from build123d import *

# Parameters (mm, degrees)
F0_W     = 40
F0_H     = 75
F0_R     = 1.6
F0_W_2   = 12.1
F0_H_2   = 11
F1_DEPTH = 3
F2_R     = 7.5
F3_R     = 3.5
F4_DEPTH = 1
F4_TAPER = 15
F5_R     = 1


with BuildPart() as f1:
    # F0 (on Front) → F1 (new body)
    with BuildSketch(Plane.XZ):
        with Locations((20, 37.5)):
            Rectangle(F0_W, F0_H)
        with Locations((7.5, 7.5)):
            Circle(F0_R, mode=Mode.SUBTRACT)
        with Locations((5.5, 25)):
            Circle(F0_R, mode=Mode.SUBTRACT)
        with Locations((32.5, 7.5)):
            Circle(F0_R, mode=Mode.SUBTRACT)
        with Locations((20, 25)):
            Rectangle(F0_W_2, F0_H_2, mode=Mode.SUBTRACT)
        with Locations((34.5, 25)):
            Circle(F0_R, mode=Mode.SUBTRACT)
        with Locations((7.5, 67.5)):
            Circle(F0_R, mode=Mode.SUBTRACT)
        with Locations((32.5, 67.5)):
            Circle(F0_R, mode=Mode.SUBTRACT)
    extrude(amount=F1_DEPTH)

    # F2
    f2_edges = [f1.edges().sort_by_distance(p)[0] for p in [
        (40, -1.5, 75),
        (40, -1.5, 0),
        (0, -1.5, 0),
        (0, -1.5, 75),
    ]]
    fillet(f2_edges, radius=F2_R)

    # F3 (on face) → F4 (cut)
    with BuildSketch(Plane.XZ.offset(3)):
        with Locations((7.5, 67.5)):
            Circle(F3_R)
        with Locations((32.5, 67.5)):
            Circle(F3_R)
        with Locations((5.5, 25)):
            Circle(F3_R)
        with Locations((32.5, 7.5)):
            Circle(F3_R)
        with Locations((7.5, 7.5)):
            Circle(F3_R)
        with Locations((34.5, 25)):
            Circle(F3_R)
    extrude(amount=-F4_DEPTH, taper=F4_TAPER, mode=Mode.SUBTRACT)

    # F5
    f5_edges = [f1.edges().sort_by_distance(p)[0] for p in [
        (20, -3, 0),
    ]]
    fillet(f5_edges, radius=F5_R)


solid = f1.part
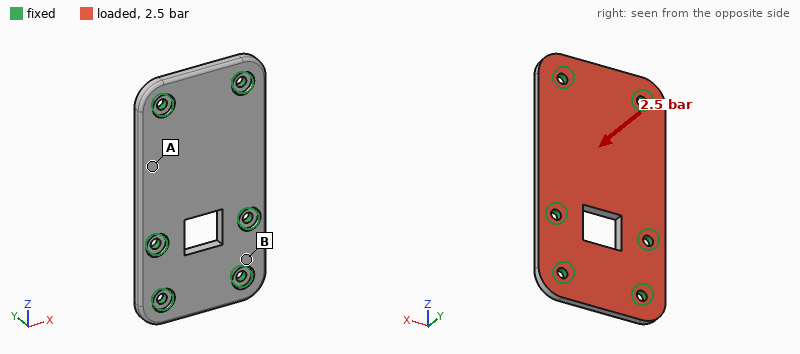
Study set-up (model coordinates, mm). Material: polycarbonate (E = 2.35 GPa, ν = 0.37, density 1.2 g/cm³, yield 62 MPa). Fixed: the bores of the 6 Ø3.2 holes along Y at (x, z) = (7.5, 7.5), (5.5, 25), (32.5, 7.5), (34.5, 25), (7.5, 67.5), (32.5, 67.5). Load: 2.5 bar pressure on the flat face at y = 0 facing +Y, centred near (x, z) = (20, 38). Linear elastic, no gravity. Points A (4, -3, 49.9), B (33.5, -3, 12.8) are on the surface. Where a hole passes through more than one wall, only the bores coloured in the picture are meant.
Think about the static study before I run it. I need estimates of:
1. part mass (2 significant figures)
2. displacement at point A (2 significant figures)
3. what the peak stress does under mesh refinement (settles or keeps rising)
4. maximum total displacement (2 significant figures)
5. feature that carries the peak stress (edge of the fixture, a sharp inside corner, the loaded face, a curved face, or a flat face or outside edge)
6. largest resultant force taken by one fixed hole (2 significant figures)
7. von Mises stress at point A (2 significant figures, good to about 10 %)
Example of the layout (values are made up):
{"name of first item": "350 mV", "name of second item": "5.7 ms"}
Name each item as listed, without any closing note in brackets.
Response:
{"part mass": "9.7 g", "displacement at point A": "0.57 mm", "what the peak stress does under mesh refinement": "keeps rising", "maximum total displacement": "0.63 mm", "feature that carries the peak stress": "edge of the fixture", "largest resultant force taken by one fixed hole": "160 N", "von Mises stress at point A": "16 MPa"}
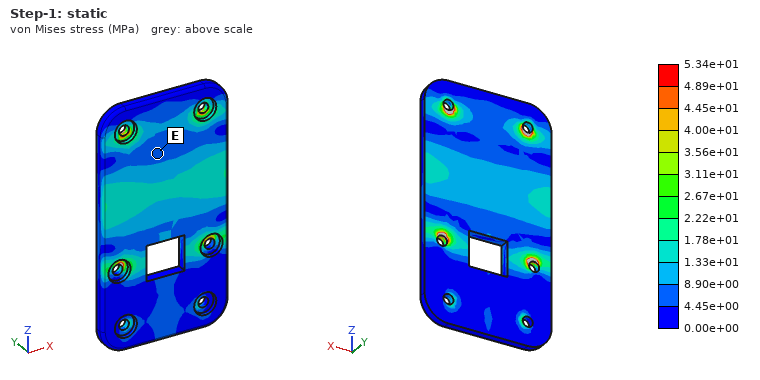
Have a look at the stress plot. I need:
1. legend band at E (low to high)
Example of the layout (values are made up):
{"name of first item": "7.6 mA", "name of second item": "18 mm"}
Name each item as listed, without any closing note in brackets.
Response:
{"legend band at E": "4.45e+00 to 8.90e+00 MPa"}
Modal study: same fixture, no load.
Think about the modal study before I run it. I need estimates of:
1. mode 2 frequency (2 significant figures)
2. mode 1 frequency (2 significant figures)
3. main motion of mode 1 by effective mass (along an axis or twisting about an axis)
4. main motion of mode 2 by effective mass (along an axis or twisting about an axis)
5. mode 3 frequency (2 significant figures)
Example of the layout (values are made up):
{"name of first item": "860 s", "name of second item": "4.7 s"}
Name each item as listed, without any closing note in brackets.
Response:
{"mode 2 frequency": "2500 Hz", "mode 1 frequency": "1900 Hz", "main motion of mode 1 by effective mass": "along Y", "main motion of mode 2 by effective mass": "twisting about Z", "mode 3 frequency": "3900 Hz"}
